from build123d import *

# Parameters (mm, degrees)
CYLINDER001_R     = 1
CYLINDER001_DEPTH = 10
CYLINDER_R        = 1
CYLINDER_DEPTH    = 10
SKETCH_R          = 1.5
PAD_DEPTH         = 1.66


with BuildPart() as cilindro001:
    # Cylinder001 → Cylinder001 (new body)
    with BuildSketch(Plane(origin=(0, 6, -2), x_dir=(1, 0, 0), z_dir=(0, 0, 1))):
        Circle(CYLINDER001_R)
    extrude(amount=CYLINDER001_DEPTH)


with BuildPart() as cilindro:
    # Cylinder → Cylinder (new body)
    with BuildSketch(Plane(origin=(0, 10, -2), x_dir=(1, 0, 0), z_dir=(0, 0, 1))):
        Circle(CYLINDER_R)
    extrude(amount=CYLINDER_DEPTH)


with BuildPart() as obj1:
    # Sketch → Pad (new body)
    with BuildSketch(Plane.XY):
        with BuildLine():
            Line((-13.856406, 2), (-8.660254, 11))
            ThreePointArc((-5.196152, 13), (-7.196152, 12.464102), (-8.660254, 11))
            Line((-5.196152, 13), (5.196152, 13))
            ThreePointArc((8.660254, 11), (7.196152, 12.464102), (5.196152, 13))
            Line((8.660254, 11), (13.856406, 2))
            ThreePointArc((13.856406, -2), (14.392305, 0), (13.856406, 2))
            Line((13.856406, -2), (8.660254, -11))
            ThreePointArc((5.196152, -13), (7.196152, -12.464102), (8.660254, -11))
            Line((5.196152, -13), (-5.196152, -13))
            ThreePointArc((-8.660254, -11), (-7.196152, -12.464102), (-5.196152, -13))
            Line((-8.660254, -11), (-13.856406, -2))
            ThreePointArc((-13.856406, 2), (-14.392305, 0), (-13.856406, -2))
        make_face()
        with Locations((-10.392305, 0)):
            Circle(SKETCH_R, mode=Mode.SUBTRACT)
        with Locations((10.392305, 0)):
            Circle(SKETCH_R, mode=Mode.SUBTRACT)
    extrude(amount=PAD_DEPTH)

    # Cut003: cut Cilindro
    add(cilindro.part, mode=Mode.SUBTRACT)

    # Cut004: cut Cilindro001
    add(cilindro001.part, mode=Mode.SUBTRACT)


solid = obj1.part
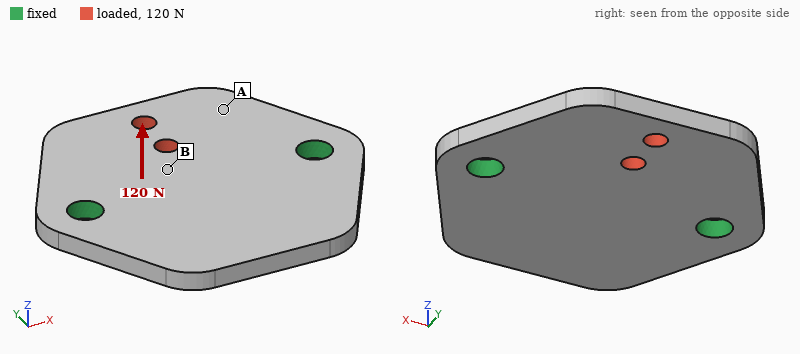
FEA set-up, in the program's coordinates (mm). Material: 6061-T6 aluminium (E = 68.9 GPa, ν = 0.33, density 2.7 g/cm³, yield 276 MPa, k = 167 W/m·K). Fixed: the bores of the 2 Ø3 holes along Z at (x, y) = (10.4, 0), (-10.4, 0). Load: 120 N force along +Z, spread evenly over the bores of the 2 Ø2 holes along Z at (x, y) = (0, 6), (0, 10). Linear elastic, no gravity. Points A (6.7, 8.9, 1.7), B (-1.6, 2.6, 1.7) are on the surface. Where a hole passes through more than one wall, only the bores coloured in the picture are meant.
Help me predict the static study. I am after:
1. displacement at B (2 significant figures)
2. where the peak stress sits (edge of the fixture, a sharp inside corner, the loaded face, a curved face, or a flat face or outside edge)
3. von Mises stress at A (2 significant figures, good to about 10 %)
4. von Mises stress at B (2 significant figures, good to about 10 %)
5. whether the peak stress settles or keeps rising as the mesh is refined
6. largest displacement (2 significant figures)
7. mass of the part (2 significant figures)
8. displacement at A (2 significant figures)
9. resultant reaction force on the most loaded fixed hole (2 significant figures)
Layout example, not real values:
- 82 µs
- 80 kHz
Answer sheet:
- 0.024 mm
- edge of the fixture
- 20 MPa
- 51 MPa
- keeps rising
- 0.10 mm
- 2.5 g
- 0.050 mm
- 60 N
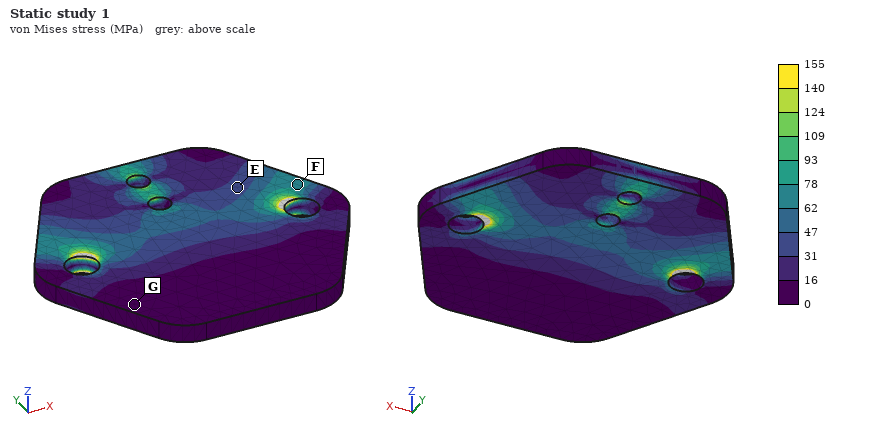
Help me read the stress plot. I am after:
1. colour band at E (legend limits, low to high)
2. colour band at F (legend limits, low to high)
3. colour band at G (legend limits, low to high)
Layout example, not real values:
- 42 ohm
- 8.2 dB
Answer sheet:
- 31 to 47 MPa
- 62 to 78 MPa
- 0 to 16 MPa
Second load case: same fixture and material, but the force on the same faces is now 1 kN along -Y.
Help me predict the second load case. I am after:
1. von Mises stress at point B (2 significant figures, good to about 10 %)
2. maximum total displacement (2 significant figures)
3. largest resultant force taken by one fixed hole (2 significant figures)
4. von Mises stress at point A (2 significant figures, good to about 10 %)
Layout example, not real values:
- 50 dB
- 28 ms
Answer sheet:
- 37 MPa
- 12 µm
- 520 N
- 20 MPa
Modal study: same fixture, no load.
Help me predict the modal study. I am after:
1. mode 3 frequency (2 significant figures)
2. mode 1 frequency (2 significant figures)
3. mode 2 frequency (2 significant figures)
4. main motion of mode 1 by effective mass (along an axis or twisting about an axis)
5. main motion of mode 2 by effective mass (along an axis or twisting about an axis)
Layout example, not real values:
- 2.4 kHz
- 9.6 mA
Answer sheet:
- 19 kHz
- 7700 Hz
- 9400 Hz
- twisting about X
- along Z
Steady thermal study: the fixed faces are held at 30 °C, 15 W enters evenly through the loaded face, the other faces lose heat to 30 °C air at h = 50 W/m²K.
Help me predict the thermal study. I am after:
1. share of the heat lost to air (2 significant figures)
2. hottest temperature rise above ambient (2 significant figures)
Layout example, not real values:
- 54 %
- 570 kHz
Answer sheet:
- 4.4 %
- 34 K
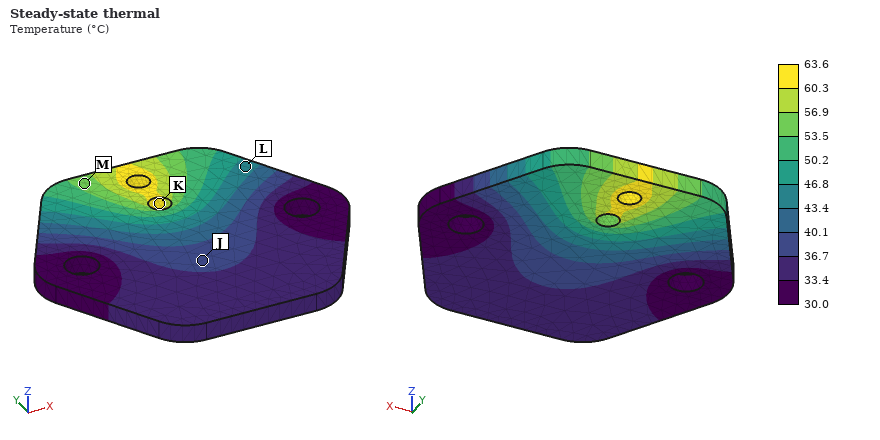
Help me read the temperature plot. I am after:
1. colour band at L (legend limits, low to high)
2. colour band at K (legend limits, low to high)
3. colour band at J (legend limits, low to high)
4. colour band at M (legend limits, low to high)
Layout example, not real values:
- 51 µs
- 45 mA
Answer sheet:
- 43.4 to 46.8 °C
- 60.3 to 63.6 °C
- 36.7 to 40.1 °C
- 53.5 to 56.9 °C
